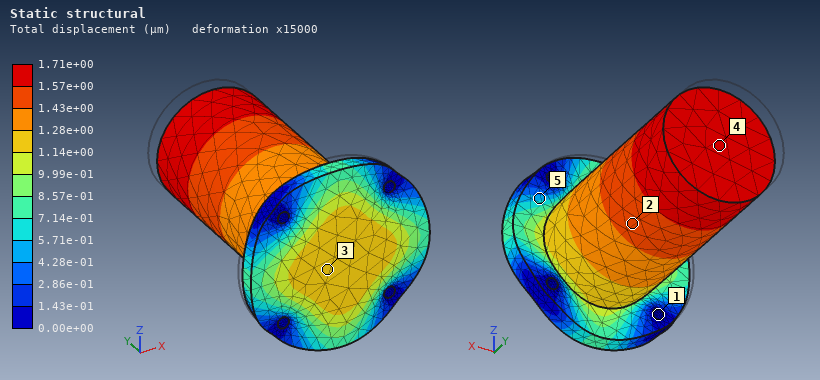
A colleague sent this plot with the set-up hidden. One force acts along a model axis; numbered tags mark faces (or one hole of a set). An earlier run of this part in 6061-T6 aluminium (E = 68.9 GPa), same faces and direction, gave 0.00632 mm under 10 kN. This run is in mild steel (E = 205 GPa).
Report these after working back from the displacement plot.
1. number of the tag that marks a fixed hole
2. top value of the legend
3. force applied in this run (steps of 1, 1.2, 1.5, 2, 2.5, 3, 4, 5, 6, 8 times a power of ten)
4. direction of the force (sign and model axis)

1
1.71e+00 µm
8 kN
-Y
